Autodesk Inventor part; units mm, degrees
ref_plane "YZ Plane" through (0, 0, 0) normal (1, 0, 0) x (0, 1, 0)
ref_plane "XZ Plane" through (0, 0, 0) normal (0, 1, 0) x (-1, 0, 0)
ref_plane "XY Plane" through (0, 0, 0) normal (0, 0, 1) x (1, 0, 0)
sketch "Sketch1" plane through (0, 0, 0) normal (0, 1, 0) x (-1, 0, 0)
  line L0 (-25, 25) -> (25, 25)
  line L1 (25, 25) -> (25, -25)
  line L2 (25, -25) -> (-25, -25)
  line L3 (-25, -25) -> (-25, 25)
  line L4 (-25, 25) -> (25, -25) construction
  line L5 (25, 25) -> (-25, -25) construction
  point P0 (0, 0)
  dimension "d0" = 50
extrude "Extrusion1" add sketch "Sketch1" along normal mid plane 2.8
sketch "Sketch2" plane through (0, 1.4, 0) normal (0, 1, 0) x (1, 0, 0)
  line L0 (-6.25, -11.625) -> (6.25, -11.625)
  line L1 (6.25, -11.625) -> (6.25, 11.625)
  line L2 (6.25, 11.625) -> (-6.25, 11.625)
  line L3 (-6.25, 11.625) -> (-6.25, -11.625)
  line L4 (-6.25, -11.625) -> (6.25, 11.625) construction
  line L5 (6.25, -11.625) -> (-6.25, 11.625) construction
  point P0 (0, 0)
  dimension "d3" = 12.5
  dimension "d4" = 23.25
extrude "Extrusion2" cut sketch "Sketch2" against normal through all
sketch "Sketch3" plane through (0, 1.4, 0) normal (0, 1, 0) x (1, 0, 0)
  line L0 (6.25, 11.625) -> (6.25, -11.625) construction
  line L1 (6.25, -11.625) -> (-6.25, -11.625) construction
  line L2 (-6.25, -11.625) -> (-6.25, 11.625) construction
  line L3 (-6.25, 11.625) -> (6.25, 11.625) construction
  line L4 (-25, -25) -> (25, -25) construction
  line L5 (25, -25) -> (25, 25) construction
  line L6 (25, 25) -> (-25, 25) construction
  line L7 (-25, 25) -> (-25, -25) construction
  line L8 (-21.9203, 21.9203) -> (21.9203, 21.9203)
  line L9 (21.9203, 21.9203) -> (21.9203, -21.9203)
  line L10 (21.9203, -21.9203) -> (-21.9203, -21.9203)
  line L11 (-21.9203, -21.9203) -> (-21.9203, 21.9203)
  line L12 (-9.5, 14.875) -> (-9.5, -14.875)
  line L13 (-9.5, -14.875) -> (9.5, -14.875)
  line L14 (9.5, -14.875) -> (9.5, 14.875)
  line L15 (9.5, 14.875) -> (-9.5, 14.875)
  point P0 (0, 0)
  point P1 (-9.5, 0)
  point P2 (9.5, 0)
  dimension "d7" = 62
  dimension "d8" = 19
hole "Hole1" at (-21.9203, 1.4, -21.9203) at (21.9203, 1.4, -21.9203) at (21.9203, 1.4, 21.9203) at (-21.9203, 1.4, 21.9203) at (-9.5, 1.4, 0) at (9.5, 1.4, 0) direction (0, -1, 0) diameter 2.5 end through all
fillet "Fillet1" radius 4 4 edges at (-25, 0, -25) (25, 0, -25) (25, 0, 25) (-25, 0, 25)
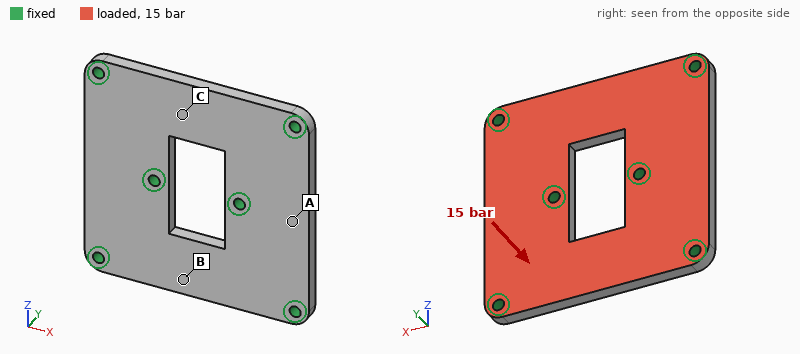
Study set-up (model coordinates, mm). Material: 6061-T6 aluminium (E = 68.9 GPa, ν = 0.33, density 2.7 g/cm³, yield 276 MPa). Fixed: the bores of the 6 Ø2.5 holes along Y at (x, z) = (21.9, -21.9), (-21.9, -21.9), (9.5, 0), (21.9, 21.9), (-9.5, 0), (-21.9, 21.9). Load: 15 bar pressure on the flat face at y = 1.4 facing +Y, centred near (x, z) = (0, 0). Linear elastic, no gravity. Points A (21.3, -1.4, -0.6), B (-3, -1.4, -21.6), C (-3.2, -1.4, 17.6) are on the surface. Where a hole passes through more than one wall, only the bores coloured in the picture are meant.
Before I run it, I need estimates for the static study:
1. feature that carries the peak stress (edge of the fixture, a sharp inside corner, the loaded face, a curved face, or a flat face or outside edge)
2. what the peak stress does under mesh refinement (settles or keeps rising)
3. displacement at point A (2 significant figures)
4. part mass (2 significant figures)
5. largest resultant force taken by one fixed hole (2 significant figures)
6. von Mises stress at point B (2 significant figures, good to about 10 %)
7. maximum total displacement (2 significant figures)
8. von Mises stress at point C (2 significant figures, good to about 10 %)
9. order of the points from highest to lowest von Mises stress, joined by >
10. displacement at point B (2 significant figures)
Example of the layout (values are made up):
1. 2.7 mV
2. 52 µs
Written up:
1. edge of the fixture
2. keeps rising
3. 23 µm
4. 16 g
5. 720 N
6. 59 MPa
7. 96 µm
8. 47 MPa
9. B > C > A
10. 82 µm
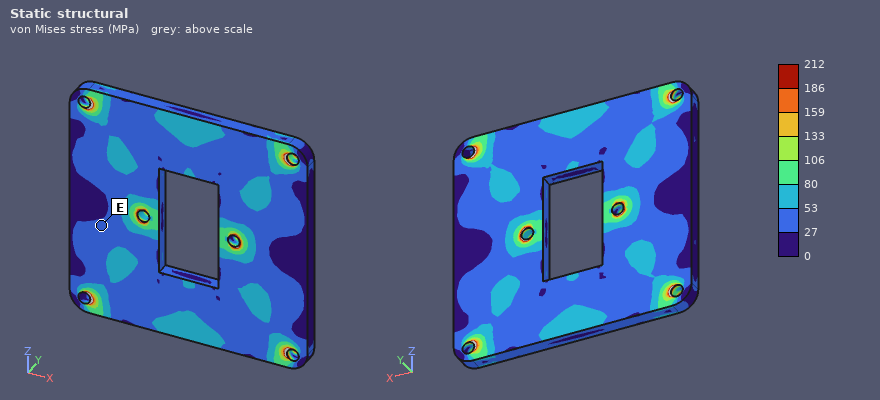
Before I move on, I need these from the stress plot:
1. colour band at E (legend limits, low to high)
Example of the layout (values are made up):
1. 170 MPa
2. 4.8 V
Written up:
1. 27 to 53 MPa
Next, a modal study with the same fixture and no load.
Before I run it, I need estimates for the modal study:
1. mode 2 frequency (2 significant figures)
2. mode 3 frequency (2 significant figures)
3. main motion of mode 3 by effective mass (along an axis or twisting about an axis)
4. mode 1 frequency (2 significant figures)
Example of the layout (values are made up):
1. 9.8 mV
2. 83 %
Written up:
1. 8900 Hz
2. 13 kHz
3. twisting about Z
4. 8600 Hz
